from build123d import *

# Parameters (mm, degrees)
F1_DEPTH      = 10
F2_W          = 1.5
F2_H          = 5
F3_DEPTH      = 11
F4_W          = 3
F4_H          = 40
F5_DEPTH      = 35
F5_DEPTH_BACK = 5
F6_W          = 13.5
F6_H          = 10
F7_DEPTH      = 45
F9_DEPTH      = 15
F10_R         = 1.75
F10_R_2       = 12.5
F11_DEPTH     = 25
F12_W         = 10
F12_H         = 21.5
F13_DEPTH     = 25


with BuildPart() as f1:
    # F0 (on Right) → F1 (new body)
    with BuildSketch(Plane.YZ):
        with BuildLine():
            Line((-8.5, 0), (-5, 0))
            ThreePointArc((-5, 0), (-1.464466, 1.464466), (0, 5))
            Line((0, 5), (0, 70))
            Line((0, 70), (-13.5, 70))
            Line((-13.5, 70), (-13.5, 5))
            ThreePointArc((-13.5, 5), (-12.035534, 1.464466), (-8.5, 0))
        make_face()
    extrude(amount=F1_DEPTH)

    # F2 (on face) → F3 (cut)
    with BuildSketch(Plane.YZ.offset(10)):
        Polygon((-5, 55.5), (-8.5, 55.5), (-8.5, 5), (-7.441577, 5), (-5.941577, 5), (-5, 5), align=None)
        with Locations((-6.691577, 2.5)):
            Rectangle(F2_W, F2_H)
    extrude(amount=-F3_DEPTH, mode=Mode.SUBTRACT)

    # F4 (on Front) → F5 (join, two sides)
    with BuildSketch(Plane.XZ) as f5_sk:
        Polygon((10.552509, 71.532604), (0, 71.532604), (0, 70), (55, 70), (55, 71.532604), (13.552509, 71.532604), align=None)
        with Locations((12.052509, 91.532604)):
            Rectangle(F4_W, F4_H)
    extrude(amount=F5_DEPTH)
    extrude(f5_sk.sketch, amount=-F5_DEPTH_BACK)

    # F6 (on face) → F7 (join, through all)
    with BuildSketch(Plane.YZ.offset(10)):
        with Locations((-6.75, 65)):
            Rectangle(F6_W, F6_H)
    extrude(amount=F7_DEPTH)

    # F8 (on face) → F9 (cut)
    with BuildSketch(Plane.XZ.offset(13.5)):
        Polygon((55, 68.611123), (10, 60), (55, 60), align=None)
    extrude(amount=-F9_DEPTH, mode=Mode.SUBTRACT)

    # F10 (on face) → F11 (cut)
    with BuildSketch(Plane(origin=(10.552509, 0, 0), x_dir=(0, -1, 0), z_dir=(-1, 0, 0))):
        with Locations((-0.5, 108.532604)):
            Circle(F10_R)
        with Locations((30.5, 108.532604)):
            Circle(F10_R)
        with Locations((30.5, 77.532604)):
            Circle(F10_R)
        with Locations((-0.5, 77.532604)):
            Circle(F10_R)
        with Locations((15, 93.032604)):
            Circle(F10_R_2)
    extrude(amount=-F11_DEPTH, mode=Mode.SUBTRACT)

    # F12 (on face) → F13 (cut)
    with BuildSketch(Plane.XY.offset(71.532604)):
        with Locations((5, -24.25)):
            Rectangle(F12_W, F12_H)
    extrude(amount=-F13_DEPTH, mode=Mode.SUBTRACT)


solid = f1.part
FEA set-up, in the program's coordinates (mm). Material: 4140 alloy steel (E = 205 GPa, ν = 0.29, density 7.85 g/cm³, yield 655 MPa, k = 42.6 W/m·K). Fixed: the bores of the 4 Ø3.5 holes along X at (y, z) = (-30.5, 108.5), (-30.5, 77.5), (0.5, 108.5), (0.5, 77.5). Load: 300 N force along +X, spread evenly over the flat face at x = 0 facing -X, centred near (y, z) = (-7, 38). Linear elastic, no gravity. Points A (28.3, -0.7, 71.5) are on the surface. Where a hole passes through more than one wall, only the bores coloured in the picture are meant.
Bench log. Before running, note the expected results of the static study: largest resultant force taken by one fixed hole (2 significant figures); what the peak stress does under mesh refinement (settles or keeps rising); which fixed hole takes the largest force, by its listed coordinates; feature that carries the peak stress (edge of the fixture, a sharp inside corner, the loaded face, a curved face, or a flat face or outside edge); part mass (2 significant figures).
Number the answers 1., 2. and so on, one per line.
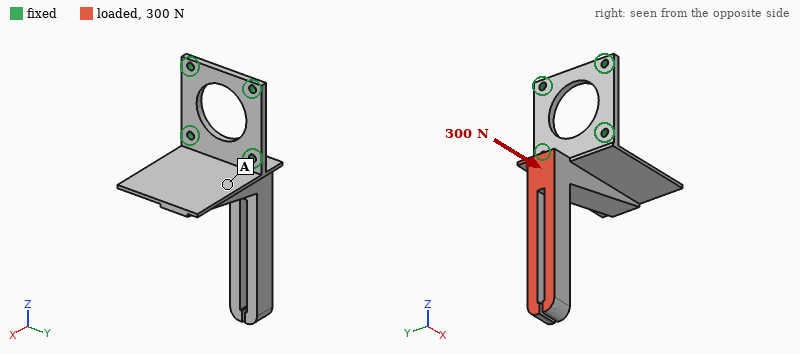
1. 210 N
2. keeps rising
3. (0.5, 77.5)
4. edge of the fixture
5. 140 g
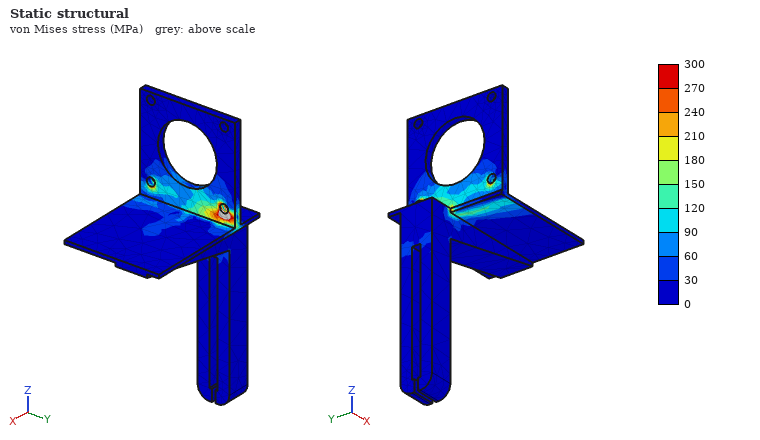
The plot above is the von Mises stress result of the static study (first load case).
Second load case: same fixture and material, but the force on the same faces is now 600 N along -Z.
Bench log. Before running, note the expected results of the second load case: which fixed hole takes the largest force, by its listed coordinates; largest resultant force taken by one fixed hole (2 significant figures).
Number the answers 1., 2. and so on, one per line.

1. (0.5, 77.5)
2. 480 N
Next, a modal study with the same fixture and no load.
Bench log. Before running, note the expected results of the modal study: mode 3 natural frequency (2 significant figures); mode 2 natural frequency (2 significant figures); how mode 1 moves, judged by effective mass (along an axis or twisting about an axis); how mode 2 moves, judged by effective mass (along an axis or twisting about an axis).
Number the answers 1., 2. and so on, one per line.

1. 1200 Hz
2. 1100 Hz
3. along X
4. along Y
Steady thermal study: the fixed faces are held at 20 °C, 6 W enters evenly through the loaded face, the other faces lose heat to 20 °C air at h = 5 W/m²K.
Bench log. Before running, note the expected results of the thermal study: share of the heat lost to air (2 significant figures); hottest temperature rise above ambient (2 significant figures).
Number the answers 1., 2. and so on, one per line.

1. 17 %
2. 51 K
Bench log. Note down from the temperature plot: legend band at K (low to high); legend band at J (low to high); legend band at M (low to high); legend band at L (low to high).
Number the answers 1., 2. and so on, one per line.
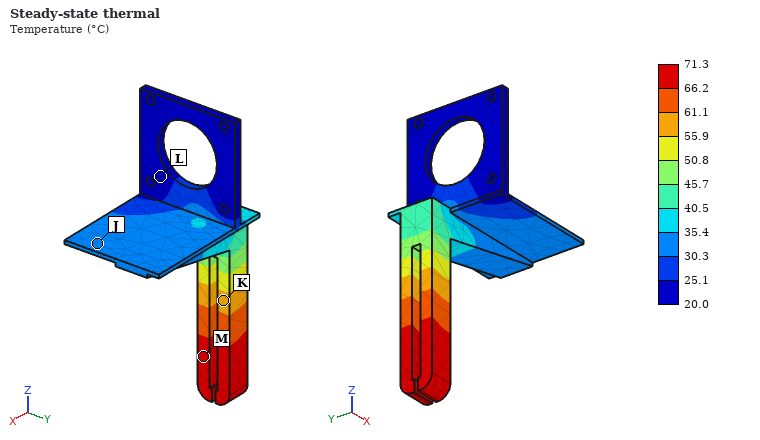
1. 55.9 to 61.1 °C
2. 30.3 to 35.4 °C
3. 66.2 to 71.3 °C
4. 20.0 to 25.1 °C
